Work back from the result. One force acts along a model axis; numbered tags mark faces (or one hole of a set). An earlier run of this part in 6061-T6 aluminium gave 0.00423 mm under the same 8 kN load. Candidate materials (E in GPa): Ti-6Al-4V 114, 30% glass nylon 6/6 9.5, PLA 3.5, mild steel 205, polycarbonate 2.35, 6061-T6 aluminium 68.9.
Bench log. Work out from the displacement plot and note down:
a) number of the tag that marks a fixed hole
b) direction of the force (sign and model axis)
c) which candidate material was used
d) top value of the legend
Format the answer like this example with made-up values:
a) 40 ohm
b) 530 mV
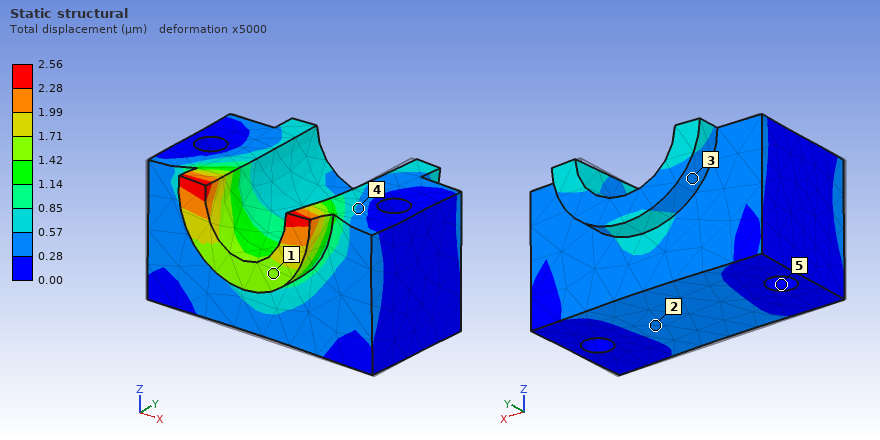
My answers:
a) 5
b) +Y
c) Ti-6Al-4V
d) 2.56 µm
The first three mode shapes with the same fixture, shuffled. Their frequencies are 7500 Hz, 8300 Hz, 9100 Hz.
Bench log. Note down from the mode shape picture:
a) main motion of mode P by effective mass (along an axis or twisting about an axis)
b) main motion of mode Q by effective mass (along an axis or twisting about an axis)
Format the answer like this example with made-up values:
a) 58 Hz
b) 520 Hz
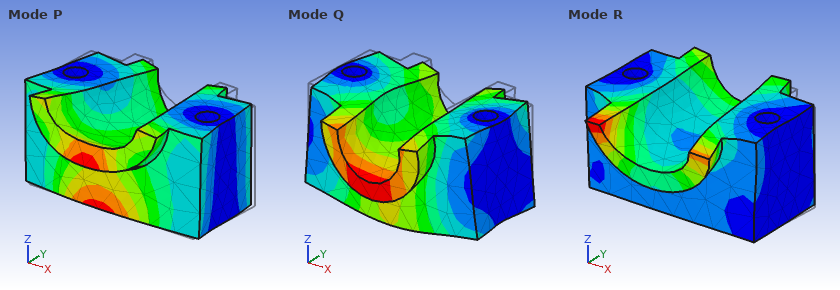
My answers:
a) along Y
b) along Z
